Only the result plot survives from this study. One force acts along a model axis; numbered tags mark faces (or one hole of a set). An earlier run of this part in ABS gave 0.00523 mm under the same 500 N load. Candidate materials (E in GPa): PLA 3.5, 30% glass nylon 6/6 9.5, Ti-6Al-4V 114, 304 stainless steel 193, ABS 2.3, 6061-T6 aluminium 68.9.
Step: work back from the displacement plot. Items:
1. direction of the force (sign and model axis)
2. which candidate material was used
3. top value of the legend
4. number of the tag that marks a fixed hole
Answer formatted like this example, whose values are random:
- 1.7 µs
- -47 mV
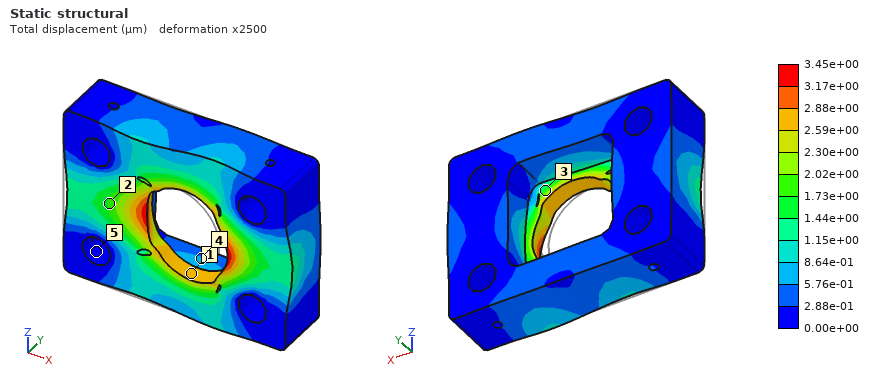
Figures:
- +X
- PLA
- 3.45e+00 µm
- 5
